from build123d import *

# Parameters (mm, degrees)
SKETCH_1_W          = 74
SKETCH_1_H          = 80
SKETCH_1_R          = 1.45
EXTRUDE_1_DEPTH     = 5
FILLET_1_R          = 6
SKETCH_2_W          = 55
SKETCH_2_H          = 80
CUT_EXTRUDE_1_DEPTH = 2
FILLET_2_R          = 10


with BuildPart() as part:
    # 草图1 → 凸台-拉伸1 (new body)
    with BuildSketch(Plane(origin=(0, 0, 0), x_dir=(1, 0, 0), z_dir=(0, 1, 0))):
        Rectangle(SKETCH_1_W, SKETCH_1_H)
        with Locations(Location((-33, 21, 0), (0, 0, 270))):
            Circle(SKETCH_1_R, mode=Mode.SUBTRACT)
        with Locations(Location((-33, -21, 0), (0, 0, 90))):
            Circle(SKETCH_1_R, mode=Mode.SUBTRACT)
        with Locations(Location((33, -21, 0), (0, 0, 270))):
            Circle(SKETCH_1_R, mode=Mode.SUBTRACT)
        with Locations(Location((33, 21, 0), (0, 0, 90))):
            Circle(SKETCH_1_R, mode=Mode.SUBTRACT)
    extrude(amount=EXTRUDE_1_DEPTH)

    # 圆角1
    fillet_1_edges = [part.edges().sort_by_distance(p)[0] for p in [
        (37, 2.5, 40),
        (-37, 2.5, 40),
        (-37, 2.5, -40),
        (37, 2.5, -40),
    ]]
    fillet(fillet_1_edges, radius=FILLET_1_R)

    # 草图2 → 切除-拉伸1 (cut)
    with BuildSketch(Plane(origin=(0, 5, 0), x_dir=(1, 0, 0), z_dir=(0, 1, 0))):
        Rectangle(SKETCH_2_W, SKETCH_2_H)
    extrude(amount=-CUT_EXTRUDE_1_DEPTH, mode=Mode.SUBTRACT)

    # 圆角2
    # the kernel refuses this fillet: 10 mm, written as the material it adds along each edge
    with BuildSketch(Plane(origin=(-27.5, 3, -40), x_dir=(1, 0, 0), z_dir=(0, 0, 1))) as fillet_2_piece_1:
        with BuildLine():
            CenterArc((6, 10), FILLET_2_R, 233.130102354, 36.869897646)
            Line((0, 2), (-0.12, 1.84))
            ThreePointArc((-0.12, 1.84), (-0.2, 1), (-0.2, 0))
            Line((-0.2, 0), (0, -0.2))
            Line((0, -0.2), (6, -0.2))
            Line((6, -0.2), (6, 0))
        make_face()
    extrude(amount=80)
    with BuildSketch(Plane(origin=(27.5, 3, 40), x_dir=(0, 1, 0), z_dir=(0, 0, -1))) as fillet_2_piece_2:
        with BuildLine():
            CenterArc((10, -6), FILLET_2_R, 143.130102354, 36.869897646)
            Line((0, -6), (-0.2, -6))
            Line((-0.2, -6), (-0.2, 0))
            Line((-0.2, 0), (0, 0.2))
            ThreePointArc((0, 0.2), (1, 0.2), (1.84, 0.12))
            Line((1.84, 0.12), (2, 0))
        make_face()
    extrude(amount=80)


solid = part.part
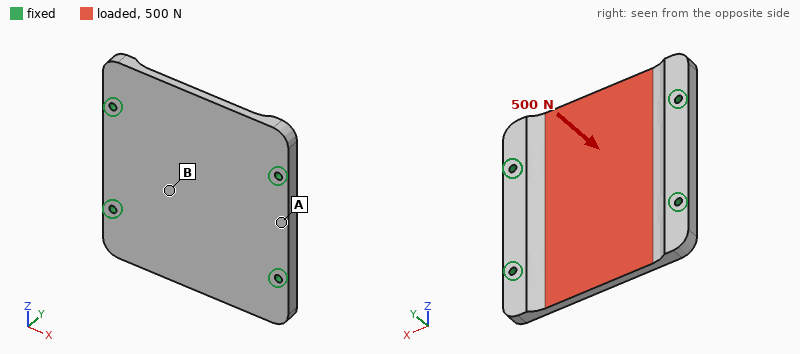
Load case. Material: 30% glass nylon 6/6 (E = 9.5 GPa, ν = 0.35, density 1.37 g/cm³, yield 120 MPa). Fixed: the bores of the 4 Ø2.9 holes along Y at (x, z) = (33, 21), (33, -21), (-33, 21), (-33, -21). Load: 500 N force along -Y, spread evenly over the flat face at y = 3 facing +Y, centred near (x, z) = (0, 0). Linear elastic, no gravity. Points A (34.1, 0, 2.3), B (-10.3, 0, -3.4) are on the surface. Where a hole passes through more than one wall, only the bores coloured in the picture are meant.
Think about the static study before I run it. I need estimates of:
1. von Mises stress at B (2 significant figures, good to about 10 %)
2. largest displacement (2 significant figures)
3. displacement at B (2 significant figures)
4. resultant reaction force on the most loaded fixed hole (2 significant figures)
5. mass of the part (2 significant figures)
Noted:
8.9 MPa
0.27 mm
0.18 mm
190 N
29 g
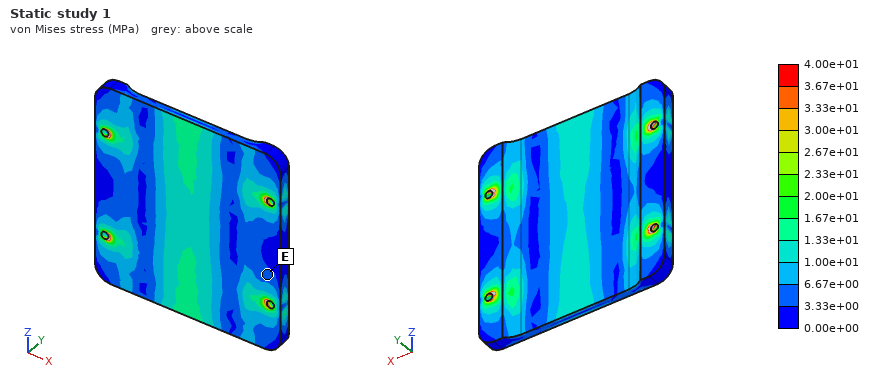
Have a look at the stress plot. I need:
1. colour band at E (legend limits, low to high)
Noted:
3.33e+00 to 6.67e+00 MPa
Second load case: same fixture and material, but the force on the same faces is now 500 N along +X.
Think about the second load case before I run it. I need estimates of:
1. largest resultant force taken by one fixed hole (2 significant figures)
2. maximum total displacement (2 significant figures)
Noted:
130 N
8.2 µm
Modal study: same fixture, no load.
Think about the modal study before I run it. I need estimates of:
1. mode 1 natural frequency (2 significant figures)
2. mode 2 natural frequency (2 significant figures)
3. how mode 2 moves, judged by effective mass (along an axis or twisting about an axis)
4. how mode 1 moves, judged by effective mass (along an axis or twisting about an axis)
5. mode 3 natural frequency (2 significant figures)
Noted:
2100 Hz
2300 Hz
twisting about X
along Y
2800 Hz
